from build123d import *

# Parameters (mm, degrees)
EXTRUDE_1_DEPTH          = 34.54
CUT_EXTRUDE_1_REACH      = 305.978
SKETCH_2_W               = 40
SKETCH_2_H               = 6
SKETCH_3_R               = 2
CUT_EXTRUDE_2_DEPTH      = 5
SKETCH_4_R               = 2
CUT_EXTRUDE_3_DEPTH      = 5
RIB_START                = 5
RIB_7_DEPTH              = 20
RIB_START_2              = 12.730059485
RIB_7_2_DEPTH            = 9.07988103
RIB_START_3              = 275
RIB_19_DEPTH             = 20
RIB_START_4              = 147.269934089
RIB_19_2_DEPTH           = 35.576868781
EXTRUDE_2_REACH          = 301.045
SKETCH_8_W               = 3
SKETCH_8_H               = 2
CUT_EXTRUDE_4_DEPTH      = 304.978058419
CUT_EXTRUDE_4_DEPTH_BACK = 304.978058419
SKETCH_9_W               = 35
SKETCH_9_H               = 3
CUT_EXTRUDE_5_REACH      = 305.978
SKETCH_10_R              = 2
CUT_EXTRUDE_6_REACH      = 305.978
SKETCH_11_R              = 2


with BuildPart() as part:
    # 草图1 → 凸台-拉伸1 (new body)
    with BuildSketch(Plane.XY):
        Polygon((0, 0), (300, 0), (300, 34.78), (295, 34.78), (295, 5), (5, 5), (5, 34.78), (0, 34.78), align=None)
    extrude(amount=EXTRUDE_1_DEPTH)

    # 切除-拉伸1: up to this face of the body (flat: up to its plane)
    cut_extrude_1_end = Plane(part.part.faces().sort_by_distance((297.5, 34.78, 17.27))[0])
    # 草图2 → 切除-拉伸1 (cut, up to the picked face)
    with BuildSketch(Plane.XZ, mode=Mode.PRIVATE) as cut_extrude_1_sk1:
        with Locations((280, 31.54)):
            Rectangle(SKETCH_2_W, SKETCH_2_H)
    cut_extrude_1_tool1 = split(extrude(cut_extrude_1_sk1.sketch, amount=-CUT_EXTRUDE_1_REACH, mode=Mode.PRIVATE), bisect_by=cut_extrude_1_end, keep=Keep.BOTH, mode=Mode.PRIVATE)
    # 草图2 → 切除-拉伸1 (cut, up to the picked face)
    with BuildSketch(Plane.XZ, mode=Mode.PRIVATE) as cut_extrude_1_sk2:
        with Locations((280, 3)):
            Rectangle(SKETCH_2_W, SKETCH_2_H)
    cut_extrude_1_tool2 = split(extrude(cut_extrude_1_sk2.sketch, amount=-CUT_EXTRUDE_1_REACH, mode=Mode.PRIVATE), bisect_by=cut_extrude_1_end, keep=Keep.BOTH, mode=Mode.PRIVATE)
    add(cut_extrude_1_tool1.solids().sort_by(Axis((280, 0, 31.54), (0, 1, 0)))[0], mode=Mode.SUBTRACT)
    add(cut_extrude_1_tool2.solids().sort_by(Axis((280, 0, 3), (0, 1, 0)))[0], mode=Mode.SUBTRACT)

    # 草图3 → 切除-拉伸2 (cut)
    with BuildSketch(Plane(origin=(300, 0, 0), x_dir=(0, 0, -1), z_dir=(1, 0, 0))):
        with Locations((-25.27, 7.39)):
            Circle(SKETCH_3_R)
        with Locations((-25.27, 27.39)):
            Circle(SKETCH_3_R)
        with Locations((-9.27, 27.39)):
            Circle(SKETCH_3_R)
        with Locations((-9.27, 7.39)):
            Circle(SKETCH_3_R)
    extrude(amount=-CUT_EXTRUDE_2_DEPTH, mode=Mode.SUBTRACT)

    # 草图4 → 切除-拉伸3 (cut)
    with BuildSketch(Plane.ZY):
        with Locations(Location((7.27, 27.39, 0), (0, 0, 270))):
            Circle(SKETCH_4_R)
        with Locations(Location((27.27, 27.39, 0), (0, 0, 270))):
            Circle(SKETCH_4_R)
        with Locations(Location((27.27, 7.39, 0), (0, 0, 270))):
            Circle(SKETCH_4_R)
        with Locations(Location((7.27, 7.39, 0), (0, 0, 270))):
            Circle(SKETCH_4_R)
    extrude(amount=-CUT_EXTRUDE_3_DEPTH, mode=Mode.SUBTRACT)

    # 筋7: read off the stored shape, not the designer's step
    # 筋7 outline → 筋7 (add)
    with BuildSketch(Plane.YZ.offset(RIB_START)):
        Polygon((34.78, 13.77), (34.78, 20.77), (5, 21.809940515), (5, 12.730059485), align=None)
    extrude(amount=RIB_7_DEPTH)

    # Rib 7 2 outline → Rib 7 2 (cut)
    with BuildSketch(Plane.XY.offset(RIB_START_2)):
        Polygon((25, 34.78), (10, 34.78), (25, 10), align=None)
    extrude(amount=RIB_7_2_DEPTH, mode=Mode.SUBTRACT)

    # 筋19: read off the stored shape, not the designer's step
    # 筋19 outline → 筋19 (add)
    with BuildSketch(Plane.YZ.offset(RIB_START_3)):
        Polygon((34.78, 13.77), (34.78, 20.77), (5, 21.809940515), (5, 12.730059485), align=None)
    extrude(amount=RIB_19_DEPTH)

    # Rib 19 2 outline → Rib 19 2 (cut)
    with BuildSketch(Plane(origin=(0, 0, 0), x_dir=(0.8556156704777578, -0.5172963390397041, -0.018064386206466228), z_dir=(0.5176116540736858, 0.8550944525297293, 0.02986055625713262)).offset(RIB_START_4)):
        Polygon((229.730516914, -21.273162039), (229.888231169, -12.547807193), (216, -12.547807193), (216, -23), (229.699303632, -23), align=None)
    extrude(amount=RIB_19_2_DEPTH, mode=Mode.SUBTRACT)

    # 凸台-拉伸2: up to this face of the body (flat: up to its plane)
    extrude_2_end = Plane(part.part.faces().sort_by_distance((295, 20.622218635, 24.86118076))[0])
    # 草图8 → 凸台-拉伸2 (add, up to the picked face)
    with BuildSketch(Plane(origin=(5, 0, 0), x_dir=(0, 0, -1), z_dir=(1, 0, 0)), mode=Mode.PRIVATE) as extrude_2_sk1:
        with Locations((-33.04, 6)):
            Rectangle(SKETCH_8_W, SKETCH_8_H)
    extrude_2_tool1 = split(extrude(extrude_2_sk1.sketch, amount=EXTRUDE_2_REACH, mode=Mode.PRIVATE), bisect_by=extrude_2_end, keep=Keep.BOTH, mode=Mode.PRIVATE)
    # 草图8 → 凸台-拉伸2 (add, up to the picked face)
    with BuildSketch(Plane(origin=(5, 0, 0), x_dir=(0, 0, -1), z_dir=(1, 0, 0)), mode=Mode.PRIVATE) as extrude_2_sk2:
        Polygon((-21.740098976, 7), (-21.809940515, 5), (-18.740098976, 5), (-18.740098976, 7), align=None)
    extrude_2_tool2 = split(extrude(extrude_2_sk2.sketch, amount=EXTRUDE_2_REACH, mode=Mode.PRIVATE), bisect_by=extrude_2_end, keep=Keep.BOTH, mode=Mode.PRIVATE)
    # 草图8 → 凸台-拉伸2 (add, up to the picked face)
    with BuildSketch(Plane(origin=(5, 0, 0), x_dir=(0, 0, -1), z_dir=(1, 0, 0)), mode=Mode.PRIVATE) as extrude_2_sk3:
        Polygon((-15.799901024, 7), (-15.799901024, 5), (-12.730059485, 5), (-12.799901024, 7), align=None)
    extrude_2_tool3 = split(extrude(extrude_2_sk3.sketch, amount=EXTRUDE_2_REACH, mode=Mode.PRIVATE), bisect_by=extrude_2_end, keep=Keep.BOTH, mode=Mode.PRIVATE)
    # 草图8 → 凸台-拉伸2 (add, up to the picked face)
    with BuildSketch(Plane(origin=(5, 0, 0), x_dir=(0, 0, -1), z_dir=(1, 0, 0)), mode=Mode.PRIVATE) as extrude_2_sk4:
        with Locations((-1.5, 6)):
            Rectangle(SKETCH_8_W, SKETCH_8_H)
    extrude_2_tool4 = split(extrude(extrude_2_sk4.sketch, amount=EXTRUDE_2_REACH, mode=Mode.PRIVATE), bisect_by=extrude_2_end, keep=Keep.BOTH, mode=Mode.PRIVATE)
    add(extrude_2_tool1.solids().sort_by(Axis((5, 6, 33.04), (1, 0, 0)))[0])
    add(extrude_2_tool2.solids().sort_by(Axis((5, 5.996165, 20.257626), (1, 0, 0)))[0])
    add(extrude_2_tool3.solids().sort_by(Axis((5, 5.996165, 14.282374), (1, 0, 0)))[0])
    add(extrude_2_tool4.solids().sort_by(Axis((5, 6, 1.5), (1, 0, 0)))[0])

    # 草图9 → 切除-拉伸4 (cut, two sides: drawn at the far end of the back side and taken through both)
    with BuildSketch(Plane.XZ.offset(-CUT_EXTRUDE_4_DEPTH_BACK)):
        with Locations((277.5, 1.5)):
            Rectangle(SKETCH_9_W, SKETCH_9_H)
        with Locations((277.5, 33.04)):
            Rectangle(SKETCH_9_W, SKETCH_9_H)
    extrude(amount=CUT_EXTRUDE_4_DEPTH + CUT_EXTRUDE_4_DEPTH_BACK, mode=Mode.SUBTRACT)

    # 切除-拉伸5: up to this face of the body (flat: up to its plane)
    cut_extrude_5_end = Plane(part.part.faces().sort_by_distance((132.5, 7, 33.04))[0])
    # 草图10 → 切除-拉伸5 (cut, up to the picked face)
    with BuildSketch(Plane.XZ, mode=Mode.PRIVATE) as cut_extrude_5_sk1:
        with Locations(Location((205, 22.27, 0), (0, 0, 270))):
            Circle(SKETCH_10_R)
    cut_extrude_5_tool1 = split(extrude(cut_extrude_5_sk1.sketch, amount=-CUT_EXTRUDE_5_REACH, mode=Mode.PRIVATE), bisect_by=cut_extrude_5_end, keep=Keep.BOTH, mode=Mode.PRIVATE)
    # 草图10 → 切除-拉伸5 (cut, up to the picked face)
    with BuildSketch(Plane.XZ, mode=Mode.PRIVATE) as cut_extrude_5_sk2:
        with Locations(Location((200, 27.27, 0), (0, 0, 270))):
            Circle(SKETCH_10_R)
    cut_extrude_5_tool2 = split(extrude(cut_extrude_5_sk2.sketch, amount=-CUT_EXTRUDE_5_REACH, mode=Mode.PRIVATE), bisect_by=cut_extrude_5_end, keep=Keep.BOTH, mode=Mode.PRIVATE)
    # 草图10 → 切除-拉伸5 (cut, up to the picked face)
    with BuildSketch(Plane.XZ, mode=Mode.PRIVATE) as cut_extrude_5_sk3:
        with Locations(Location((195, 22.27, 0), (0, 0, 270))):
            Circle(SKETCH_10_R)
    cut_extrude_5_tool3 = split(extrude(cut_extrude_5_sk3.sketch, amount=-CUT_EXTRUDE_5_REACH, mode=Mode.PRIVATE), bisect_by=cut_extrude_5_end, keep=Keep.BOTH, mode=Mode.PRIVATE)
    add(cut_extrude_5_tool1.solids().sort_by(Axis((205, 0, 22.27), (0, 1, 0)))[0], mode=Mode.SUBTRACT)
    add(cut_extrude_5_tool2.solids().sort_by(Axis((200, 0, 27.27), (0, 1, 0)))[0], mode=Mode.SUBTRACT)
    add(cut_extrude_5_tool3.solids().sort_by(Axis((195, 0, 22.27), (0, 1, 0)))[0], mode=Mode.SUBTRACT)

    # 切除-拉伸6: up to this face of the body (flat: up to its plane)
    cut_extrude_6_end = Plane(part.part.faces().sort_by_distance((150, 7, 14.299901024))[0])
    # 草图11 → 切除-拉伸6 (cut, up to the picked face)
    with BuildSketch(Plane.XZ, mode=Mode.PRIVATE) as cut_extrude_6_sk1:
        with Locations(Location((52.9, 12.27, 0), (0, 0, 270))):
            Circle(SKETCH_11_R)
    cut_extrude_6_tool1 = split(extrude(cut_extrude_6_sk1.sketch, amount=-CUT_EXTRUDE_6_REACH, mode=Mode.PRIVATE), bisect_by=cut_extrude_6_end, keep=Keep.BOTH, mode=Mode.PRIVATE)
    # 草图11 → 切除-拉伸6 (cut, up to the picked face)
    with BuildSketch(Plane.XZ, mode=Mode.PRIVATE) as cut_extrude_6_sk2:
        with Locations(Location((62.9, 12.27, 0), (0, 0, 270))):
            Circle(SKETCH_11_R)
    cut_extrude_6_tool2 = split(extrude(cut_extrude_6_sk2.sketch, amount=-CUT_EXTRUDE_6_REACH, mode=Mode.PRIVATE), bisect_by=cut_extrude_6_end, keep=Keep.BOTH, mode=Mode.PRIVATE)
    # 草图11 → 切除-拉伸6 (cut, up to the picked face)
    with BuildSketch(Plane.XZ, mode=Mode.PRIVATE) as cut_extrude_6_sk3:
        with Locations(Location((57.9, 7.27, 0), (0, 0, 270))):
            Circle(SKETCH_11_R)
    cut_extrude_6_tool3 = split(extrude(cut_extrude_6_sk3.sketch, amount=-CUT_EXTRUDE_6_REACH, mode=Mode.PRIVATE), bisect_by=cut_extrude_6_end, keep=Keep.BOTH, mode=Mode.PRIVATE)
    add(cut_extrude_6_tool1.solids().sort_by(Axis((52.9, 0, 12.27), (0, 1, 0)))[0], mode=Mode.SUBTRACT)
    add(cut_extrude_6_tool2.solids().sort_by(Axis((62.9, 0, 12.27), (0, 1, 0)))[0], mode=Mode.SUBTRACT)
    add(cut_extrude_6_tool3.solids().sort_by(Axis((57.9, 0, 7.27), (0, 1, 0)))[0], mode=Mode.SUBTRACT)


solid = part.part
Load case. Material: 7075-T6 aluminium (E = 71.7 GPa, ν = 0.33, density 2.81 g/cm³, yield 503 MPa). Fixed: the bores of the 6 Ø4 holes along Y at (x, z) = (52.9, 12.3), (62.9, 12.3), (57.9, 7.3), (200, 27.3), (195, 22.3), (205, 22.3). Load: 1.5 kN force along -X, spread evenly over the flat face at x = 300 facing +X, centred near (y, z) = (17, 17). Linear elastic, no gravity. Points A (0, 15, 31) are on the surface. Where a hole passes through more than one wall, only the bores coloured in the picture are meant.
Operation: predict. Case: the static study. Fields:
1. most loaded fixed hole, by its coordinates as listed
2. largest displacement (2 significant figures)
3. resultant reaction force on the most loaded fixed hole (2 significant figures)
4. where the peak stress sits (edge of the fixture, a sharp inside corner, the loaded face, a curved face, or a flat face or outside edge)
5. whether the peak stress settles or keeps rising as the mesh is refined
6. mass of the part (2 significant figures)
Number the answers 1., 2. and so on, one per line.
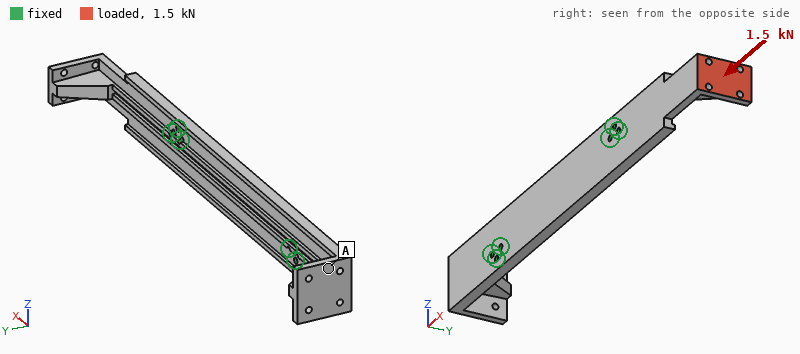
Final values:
1. (205, 22.3)
2. 2.8 mm
3. 1.4 kN
4. edge of the fixture
5. keeps rising
6. 200 g
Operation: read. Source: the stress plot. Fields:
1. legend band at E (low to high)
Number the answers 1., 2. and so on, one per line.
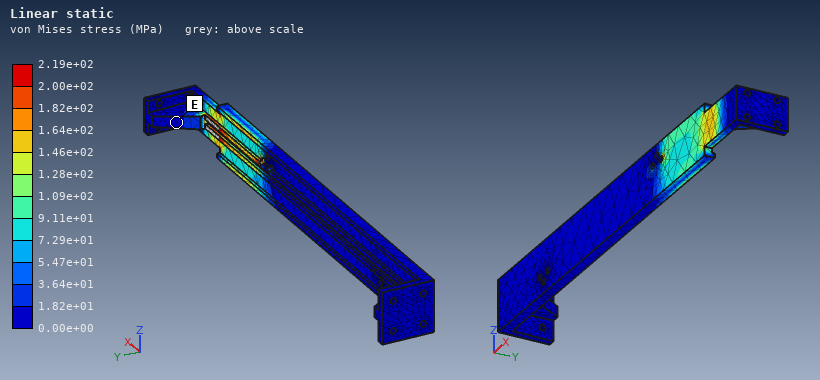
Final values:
1. 0.00e+00 to 1.82e+01 MPa
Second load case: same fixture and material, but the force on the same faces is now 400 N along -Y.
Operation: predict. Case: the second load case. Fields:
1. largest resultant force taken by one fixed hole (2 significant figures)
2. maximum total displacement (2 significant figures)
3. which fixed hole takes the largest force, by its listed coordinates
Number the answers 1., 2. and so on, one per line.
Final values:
1. 2.1 kN
2. 3.2 mm
3. (205, 22.3)
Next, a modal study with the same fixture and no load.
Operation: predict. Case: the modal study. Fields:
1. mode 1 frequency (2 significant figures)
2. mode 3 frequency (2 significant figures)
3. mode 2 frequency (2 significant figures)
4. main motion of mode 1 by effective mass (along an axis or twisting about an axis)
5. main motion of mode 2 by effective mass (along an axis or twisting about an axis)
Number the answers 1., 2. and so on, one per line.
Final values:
1. 390 Hz
2. 1100 Hz
3. 870 Hz
4. along Y
5. along Y
